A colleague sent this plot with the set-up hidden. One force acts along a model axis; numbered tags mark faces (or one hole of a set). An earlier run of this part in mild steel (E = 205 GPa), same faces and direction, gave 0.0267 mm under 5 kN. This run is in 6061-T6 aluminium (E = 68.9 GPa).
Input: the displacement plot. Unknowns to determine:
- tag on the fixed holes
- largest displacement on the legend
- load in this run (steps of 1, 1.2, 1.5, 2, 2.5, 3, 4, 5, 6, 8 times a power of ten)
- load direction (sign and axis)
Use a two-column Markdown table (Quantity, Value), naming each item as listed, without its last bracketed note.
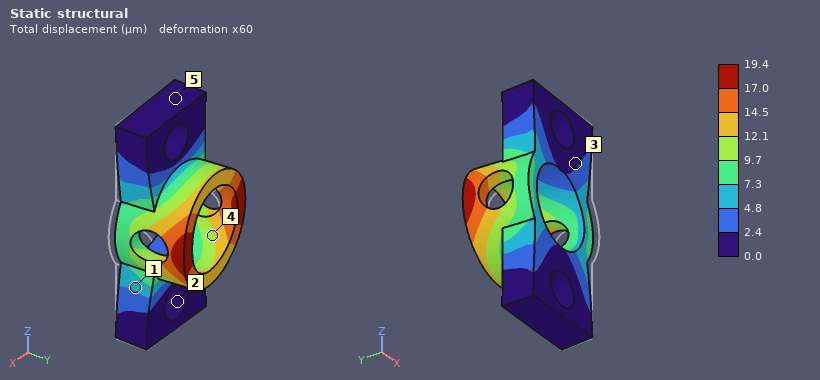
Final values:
| Quantity | Value |
|---|---|
| tag on the fixed holes | 2 |
| largest displacement on the legend | 19.4 µm |
| load in this run | 1.2 kN |
| load direction | -X |
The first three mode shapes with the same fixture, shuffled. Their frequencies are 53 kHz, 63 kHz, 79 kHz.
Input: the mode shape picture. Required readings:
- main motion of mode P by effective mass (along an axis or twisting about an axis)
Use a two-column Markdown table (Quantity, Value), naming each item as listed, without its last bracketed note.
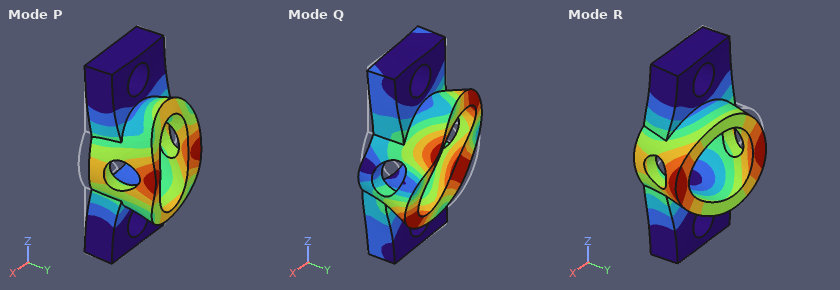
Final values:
| Quantity | Value |
|---|---|
| main motion of mode P by effective mass | along Y |
